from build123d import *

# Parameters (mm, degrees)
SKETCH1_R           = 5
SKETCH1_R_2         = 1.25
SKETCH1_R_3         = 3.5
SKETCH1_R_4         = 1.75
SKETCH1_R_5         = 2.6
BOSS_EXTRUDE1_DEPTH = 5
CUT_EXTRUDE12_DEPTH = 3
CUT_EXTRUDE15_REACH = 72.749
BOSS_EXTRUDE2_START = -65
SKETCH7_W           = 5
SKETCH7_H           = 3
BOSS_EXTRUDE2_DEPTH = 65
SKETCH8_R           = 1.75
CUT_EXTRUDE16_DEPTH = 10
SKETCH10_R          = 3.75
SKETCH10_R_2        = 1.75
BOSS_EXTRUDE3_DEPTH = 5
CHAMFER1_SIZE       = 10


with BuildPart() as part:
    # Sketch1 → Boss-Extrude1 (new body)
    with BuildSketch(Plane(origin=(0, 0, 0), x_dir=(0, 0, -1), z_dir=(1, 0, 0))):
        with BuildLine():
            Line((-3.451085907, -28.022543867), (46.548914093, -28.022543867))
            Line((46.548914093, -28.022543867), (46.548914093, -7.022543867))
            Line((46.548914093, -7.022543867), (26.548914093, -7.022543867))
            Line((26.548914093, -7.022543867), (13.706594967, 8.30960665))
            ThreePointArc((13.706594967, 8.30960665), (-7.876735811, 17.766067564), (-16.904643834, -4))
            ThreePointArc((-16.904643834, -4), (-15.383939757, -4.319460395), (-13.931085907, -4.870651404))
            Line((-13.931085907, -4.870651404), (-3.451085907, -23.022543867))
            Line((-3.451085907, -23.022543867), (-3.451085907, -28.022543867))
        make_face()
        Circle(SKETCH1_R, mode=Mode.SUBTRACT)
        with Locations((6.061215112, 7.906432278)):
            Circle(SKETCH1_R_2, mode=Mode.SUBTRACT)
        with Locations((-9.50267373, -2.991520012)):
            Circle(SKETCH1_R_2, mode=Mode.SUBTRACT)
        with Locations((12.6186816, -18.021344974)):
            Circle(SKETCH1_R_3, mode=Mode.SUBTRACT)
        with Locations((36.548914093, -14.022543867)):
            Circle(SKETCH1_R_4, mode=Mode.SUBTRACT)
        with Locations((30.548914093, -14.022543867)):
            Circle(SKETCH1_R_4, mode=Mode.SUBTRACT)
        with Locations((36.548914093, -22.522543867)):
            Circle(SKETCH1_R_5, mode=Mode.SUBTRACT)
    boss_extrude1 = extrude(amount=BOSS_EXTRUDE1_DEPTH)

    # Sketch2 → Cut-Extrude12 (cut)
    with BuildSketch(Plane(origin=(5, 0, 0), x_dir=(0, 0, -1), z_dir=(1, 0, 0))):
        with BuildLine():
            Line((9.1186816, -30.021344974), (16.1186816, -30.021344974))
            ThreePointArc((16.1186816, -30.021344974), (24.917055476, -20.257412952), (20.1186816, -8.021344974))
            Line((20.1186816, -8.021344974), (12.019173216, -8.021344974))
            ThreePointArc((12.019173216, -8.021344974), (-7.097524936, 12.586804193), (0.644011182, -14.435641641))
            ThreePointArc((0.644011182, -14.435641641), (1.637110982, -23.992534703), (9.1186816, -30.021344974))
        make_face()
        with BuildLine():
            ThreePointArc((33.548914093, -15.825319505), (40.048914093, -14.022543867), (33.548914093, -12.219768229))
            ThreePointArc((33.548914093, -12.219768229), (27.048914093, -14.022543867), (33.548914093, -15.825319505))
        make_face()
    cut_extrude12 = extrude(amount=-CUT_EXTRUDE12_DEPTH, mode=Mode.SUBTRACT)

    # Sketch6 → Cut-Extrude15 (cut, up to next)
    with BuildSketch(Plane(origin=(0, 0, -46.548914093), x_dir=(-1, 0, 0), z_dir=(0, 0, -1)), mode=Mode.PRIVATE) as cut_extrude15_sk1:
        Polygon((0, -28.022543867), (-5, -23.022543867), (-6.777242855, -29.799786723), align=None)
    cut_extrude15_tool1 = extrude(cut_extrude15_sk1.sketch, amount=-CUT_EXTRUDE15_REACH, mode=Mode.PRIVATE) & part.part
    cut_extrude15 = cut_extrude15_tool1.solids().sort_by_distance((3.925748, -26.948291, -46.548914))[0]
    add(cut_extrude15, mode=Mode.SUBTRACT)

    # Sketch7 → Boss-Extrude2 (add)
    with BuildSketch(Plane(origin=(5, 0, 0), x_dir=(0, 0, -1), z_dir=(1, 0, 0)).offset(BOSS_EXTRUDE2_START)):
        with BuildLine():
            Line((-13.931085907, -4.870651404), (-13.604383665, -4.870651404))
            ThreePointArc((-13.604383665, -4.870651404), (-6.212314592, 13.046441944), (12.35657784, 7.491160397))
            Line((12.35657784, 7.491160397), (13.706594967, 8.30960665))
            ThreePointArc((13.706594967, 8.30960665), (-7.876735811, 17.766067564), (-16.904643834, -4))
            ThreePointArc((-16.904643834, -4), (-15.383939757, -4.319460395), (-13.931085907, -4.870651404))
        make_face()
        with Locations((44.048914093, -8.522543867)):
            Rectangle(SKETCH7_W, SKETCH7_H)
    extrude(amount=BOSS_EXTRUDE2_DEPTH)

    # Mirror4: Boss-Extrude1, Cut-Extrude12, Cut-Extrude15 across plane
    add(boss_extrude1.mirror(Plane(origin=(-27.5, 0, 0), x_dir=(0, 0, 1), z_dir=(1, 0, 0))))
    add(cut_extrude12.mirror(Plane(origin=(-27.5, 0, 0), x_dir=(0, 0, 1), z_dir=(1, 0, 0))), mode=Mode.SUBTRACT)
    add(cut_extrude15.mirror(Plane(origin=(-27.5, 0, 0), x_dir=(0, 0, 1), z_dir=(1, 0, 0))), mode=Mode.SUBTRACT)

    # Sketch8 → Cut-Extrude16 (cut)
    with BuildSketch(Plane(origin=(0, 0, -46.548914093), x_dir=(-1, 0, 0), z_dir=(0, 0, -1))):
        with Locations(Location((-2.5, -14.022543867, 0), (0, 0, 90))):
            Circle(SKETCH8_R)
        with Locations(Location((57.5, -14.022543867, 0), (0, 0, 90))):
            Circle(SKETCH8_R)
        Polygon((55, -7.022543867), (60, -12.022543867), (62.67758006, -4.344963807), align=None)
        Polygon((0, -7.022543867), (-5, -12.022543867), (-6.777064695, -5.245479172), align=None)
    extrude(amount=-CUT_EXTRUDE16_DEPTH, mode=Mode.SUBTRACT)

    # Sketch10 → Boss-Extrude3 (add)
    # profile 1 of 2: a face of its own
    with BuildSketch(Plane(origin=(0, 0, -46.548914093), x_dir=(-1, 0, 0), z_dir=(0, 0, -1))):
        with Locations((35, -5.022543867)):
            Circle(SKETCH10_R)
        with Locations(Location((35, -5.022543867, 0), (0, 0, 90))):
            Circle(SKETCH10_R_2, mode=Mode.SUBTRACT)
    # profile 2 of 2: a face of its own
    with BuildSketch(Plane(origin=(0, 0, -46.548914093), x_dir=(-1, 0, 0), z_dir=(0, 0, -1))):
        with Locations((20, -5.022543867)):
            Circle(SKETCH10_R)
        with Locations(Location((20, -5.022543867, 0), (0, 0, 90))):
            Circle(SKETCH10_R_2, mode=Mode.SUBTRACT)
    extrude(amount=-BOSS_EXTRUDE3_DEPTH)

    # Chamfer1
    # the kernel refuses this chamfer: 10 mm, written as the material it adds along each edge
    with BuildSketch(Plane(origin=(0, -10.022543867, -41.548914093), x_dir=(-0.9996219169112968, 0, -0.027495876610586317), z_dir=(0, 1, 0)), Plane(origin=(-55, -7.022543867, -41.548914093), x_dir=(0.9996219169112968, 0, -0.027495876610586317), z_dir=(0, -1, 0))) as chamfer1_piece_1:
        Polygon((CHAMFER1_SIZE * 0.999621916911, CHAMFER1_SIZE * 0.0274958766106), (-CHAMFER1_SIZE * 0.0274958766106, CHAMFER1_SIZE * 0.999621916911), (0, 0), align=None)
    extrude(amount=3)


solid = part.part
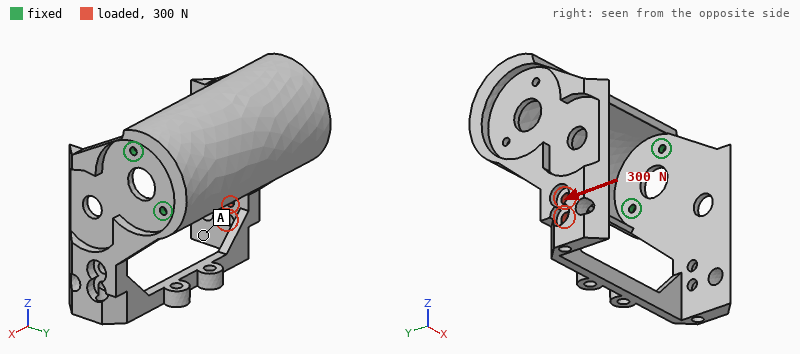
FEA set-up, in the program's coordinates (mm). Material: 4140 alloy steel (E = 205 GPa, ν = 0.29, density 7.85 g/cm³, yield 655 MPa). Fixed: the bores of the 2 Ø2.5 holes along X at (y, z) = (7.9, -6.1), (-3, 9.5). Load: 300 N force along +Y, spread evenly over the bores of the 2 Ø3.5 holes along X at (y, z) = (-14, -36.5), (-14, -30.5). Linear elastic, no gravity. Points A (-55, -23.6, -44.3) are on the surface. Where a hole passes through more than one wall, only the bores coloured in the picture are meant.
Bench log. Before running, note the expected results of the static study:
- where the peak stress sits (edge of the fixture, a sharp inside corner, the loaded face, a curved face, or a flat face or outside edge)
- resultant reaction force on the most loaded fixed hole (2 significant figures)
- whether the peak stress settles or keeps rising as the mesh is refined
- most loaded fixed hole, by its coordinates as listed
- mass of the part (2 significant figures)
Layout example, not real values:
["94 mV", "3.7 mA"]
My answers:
["edge of the fixture", "770 N", "keeps rising", "(7.9, -6.1)", "170 g"]
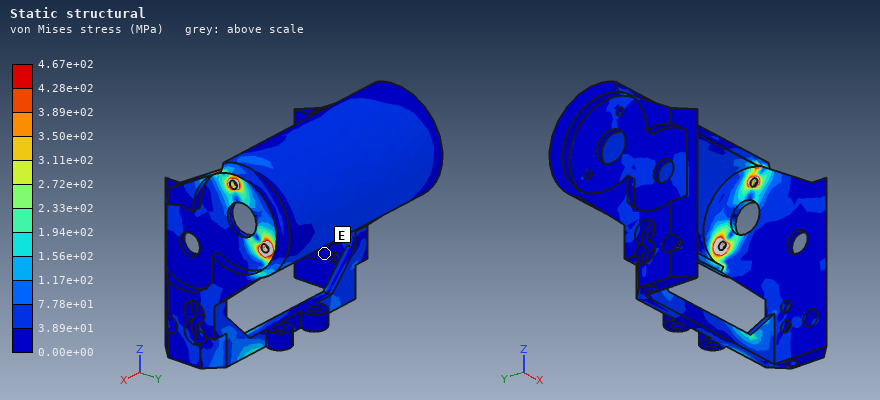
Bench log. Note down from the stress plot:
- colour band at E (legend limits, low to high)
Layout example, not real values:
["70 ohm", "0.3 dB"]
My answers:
["0.00e+00 to 3.89e+01 MPa"]
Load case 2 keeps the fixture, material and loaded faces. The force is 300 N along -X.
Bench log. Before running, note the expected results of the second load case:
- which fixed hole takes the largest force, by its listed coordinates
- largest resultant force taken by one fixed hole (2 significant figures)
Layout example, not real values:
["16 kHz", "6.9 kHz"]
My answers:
["(7.9, -6.1)", "380 N"]
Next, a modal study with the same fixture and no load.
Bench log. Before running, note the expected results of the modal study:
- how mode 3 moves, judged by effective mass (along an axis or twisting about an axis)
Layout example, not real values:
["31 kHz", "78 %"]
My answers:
["along X"]
